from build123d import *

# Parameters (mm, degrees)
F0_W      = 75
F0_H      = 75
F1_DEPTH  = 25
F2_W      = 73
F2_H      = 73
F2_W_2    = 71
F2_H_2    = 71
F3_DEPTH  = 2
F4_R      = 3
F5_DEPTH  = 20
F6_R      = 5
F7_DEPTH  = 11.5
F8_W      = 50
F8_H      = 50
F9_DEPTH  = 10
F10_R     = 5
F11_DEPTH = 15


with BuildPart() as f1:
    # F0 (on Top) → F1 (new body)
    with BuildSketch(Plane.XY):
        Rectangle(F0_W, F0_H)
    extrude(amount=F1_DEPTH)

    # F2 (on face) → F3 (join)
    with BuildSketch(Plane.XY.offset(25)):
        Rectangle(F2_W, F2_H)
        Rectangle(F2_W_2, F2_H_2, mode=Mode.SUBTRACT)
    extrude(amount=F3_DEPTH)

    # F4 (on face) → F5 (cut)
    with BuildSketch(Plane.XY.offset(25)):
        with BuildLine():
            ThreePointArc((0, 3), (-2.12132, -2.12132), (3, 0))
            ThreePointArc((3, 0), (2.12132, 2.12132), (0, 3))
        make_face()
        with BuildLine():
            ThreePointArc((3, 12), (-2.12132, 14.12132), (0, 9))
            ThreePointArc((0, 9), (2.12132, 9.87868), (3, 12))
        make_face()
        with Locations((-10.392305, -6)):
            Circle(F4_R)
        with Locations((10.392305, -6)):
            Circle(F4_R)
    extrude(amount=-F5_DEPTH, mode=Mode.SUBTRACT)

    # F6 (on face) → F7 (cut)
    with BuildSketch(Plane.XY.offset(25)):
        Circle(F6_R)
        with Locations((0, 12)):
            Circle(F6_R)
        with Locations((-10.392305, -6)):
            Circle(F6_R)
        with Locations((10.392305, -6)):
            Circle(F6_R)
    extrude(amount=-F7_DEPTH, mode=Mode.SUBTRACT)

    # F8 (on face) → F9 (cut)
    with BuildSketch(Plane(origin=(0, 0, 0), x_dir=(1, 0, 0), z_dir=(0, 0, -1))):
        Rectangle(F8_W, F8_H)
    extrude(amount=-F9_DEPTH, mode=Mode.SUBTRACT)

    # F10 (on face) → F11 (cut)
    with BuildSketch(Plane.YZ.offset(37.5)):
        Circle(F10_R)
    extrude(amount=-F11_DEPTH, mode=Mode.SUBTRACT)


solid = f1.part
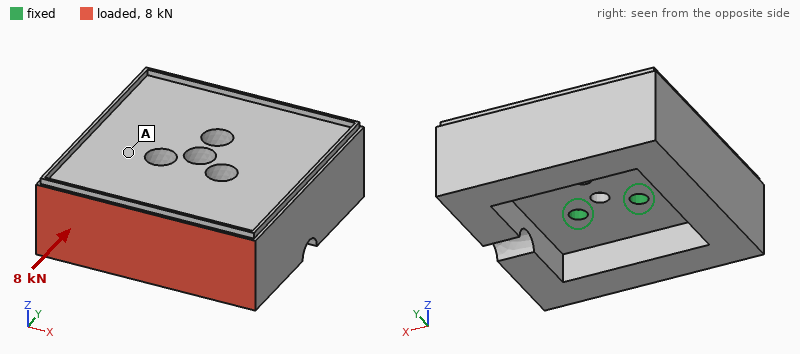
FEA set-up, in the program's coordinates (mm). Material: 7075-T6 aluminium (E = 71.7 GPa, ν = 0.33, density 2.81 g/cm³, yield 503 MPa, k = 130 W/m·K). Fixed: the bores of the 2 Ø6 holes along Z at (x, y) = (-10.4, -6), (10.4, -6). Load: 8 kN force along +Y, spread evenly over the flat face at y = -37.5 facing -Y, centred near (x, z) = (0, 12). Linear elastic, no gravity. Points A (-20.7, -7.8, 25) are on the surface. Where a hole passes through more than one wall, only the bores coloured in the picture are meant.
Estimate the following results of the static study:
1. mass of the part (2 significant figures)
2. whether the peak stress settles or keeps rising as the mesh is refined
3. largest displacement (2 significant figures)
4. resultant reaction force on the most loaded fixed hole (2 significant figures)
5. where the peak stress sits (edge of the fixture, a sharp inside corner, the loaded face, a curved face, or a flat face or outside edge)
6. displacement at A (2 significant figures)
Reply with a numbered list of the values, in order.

1. 310 g
2. keeps rising
3. 29 µm
4. 4.0 kN
5. edge of the fixture
6. 13 µm
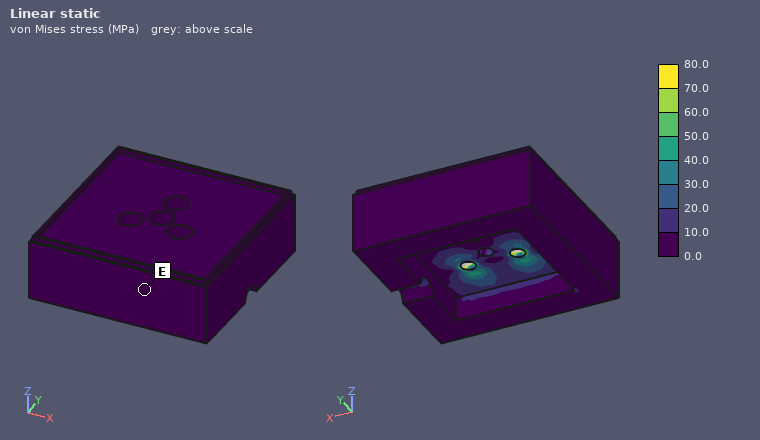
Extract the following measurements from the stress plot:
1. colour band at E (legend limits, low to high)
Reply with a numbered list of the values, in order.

1. 0.0 to 10.0 MPa
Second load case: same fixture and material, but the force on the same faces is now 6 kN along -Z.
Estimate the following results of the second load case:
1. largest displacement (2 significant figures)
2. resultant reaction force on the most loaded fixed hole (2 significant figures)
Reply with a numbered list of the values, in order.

1. 0.71 mm
2. 3.0 kN
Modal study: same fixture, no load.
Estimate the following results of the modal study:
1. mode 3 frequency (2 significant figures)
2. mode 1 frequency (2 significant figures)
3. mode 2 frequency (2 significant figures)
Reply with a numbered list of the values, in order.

1. 3300 Hz
2. 1200 Hz
3. 3200 Hz
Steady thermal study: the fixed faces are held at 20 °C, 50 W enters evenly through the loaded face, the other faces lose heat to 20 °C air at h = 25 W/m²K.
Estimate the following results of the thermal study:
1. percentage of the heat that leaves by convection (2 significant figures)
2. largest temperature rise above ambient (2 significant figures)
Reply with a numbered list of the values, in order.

1. 10 %
2. 17 K
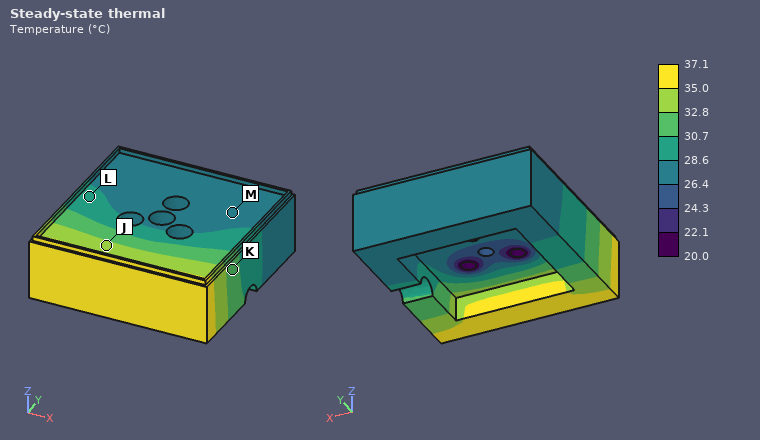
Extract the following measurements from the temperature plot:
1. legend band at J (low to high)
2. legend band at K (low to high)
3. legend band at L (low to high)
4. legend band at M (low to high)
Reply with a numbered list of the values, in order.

1. 32.8 to 35.0 °C
2. 30.7 to 32.8 °C
3. 28.6 to 30.7 °C
4. 26.4 to 28.6 °C
